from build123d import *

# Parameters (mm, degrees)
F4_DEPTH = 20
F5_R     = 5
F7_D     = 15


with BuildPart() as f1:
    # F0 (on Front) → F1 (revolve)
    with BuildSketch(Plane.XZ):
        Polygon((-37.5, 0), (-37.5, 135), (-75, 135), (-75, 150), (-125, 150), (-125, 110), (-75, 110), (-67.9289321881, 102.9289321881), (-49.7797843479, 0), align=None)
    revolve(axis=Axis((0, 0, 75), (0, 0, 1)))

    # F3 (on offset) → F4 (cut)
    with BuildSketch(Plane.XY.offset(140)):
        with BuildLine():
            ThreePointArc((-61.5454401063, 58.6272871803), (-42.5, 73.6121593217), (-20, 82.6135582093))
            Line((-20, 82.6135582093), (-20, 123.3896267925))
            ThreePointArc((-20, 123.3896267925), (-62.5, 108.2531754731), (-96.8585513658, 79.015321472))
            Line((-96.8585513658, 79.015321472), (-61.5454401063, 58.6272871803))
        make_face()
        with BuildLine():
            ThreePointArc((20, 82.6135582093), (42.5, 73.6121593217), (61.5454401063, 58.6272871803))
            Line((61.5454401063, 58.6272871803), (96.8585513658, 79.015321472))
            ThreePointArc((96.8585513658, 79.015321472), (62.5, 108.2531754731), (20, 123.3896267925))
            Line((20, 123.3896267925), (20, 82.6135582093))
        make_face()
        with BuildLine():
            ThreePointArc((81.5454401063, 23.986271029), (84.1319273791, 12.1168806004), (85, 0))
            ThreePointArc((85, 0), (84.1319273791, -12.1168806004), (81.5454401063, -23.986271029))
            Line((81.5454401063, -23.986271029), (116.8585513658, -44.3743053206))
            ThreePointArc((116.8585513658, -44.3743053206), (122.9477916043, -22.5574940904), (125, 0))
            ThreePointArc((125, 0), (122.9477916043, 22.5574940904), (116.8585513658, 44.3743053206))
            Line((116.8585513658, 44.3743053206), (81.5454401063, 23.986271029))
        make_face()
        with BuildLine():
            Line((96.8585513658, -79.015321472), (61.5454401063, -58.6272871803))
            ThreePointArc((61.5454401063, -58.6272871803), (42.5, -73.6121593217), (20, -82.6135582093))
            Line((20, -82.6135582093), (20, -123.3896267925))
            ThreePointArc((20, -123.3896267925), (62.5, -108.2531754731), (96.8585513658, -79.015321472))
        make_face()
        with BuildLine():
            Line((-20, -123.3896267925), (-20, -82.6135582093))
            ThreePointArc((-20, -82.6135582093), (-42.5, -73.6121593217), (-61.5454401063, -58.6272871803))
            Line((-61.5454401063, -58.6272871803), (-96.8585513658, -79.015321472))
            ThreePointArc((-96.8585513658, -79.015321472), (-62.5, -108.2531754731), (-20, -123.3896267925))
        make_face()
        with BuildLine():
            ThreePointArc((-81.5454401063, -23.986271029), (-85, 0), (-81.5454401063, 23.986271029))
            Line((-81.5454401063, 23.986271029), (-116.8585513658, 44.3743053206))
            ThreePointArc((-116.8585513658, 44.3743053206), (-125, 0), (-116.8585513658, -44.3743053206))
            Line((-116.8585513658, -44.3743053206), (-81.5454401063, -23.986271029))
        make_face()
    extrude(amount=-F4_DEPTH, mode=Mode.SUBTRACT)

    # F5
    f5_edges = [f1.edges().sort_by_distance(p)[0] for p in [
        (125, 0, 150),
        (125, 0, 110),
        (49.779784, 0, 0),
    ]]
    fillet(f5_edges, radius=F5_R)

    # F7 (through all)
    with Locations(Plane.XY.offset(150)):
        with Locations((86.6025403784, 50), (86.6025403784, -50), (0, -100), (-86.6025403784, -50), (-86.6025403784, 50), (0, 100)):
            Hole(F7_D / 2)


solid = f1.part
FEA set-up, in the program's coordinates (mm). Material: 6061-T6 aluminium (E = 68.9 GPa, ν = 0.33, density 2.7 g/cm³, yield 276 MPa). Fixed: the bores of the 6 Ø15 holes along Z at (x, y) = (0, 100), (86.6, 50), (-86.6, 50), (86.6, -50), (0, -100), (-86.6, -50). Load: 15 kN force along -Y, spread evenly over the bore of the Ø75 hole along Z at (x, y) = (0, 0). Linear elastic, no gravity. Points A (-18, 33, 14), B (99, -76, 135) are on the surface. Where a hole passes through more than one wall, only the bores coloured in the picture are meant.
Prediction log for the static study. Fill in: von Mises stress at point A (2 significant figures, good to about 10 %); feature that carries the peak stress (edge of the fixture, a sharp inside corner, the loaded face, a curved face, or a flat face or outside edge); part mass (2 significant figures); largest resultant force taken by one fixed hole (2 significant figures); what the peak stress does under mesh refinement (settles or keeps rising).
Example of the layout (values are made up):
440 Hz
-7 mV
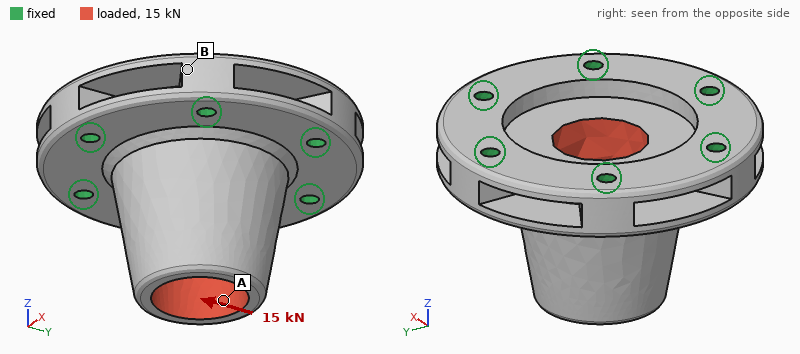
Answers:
1.7 MPa
edge of the fixture
5.3 kg
5.2 kN
keeps rising
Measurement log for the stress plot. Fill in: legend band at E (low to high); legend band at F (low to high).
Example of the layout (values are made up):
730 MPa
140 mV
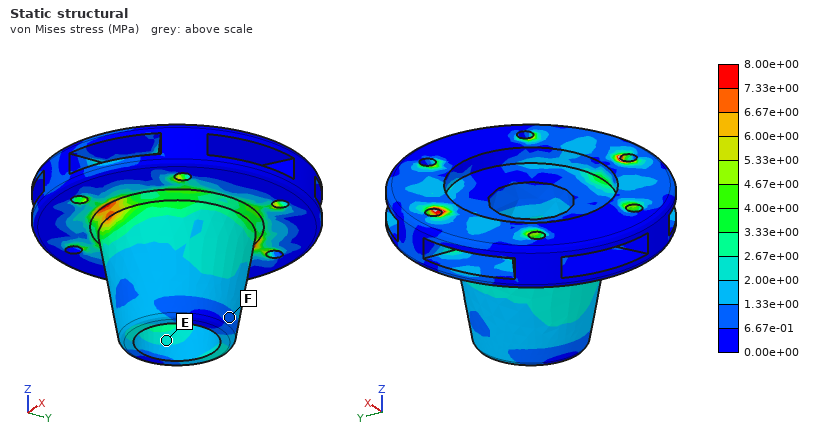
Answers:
2.00e+00 to 2.67e+00 MPa
6.67e-01 to 1.33e+00 MPa
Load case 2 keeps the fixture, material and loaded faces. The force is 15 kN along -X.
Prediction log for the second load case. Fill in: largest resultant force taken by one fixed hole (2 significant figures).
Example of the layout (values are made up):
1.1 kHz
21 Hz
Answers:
4.5 kN
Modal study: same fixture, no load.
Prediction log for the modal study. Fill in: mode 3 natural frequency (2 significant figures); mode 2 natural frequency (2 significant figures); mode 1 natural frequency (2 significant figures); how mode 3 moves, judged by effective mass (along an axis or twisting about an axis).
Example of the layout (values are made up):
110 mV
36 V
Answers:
5700 Hz
4300 Hz
4300 Hz
along Z
